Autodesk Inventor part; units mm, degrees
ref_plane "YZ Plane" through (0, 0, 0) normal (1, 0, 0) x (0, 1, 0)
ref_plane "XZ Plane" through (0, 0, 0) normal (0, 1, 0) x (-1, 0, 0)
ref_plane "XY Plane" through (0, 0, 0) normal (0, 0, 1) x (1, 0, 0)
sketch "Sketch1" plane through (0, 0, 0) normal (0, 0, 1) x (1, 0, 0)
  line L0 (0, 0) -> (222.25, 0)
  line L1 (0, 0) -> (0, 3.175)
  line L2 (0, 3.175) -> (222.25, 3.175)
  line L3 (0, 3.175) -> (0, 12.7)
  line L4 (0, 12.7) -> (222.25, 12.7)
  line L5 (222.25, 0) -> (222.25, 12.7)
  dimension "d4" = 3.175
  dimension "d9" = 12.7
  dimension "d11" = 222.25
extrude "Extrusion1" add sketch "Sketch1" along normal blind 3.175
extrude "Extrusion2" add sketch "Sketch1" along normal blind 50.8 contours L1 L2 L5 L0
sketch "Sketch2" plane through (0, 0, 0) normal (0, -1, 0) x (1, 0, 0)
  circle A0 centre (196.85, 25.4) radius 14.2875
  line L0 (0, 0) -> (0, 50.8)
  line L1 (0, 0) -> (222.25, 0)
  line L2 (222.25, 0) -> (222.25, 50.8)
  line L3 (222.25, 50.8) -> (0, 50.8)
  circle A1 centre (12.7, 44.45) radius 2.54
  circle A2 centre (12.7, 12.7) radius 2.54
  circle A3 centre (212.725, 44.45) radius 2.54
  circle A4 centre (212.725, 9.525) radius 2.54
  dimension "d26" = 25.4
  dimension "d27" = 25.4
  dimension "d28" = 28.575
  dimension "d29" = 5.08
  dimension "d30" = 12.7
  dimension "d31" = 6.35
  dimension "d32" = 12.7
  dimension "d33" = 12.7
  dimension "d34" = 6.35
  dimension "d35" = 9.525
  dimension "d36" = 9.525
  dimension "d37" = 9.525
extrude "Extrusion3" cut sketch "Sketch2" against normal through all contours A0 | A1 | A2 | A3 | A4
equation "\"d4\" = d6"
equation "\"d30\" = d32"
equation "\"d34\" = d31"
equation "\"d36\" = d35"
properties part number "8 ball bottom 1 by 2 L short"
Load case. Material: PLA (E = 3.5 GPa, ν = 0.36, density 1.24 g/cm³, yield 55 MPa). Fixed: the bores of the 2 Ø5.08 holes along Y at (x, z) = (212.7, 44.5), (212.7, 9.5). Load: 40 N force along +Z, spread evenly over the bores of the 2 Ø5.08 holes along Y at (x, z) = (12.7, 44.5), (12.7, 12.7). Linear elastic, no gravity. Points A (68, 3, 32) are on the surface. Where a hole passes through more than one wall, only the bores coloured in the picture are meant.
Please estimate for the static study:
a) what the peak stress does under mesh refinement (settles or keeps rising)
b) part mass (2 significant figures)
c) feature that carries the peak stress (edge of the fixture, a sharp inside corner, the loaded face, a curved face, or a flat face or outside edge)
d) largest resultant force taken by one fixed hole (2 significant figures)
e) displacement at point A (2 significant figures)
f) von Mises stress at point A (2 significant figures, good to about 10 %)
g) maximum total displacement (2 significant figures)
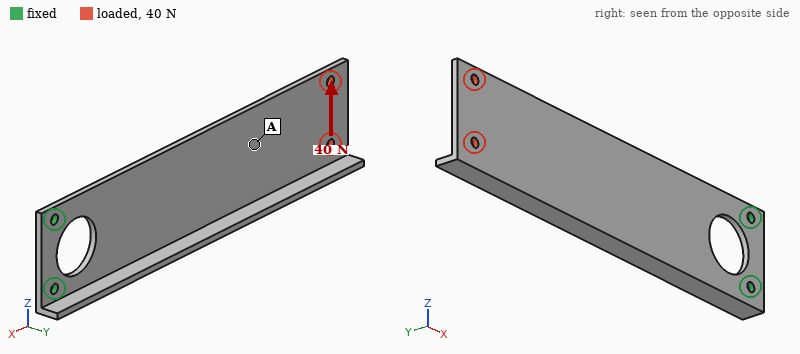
keeps rising
50 g
edge of the fixture
200 N
1.3 mm
0.92 MPa
2.5 mm
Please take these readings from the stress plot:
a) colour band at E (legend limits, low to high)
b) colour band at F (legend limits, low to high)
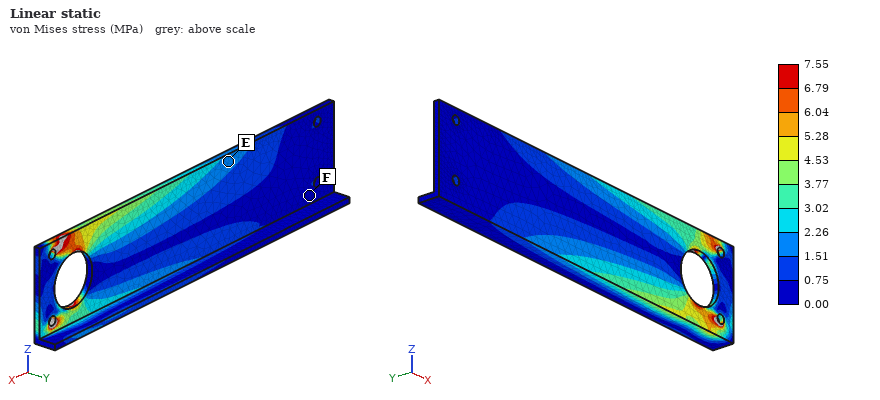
1.51 to 2.26 MPa
0.00 to 0.75 MPa
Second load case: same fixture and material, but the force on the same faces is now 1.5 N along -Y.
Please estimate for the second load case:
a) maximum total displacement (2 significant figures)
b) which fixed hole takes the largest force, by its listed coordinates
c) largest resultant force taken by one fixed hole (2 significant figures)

2.4 mm
(212.7, 44.5)
1.6 N
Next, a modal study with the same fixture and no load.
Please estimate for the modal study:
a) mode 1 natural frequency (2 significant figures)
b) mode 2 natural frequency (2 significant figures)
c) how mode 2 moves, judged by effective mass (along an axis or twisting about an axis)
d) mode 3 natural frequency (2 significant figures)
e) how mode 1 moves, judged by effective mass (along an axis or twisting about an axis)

34 Hz
140 Hz
twisting about X
220 Hz
along Y
